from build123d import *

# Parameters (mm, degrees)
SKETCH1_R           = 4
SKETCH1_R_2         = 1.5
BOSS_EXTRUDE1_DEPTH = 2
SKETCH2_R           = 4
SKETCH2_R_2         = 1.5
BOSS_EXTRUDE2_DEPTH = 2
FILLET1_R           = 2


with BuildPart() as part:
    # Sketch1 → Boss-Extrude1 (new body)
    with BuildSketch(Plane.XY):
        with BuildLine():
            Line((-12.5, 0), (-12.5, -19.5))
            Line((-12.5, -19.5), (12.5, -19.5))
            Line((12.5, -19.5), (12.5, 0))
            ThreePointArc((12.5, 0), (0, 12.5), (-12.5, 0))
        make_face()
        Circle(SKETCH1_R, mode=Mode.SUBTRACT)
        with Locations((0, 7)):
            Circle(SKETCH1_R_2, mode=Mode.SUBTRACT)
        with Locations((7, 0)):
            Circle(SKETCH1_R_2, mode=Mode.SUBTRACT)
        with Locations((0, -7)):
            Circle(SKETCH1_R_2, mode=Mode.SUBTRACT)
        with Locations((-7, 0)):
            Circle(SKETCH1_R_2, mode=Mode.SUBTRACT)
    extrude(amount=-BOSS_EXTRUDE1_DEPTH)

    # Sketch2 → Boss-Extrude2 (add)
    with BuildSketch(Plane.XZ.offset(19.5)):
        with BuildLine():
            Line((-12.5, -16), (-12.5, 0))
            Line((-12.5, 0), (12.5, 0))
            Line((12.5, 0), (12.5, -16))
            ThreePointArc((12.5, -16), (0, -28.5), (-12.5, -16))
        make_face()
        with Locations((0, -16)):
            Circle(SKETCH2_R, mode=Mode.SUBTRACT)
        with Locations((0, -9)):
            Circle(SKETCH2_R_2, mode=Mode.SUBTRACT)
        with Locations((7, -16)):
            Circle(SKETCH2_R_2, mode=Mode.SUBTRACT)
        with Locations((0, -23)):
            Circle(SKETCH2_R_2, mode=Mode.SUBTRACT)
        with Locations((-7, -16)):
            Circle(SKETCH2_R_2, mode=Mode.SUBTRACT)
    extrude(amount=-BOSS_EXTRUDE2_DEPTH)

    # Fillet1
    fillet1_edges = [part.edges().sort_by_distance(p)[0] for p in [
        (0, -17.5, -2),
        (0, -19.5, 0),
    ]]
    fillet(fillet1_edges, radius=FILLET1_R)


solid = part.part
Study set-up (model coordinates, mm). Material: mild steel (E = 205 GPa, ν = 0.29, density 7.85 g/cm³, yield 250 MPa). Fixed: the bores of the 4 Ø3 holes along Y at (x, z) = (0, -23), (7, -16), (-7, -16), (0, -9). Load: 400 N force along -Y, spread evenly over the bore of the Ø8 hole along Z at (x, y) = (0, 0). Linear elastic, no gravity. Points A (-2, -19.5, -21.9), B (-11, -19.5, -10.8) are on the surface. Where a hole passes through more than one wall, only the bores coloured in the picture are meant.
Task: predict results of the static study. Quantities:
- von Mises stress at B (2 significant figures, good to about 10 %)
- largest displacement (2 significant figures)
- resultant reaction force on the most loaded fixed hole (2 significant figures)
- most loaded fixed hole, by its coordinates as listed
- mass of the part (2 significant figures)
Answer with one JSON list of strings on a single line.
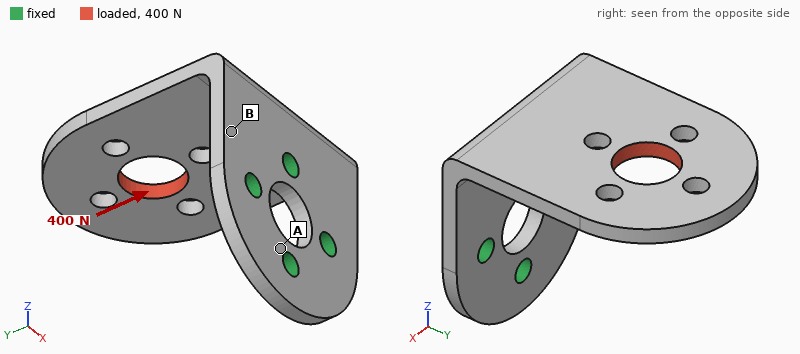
["52 MPa", "0.13 mm", "510 N", "(0, -9)", "18 g"]
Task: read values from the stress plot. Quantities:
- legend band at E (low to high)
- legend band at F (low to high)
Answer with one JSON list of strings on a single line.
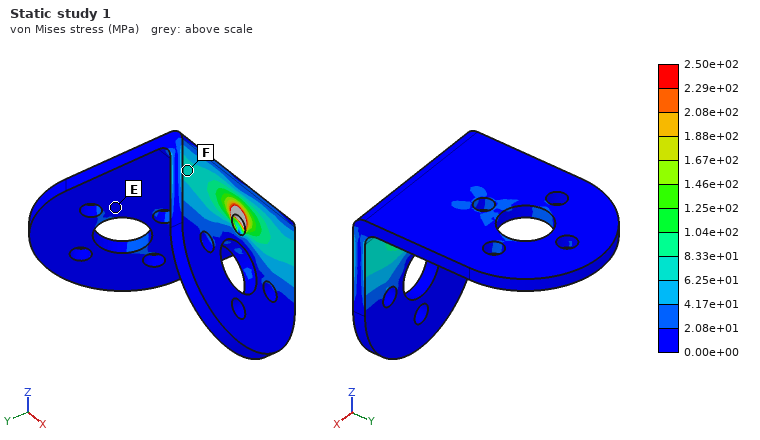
["0.00e+00 to 2.08e+01 MPa", "6.25e+01 to 8.33e+01 MPa"]
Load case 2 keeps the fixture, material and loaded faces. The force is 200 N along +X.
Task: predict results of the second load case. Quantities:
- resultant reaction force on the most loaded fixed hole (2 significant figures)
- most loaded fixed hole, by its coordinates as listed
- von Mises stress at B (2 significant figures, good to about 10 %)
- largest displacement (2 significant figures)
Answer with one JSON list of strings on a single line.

["190 N", "(0, -9)", "91 MPa", "0.12 mm"]
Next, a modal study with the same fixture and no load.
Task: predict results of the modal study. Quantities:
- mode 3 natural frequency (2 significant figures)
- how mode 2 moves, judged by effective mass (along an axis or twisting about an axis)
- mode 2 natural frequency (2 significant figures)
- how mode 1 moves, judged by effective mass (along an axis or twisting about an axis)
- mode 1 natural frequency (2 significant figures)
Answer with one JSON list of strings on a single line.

["5700 Hz", "along X", "2800 Hz", "along Z", "1600 Hz"]
